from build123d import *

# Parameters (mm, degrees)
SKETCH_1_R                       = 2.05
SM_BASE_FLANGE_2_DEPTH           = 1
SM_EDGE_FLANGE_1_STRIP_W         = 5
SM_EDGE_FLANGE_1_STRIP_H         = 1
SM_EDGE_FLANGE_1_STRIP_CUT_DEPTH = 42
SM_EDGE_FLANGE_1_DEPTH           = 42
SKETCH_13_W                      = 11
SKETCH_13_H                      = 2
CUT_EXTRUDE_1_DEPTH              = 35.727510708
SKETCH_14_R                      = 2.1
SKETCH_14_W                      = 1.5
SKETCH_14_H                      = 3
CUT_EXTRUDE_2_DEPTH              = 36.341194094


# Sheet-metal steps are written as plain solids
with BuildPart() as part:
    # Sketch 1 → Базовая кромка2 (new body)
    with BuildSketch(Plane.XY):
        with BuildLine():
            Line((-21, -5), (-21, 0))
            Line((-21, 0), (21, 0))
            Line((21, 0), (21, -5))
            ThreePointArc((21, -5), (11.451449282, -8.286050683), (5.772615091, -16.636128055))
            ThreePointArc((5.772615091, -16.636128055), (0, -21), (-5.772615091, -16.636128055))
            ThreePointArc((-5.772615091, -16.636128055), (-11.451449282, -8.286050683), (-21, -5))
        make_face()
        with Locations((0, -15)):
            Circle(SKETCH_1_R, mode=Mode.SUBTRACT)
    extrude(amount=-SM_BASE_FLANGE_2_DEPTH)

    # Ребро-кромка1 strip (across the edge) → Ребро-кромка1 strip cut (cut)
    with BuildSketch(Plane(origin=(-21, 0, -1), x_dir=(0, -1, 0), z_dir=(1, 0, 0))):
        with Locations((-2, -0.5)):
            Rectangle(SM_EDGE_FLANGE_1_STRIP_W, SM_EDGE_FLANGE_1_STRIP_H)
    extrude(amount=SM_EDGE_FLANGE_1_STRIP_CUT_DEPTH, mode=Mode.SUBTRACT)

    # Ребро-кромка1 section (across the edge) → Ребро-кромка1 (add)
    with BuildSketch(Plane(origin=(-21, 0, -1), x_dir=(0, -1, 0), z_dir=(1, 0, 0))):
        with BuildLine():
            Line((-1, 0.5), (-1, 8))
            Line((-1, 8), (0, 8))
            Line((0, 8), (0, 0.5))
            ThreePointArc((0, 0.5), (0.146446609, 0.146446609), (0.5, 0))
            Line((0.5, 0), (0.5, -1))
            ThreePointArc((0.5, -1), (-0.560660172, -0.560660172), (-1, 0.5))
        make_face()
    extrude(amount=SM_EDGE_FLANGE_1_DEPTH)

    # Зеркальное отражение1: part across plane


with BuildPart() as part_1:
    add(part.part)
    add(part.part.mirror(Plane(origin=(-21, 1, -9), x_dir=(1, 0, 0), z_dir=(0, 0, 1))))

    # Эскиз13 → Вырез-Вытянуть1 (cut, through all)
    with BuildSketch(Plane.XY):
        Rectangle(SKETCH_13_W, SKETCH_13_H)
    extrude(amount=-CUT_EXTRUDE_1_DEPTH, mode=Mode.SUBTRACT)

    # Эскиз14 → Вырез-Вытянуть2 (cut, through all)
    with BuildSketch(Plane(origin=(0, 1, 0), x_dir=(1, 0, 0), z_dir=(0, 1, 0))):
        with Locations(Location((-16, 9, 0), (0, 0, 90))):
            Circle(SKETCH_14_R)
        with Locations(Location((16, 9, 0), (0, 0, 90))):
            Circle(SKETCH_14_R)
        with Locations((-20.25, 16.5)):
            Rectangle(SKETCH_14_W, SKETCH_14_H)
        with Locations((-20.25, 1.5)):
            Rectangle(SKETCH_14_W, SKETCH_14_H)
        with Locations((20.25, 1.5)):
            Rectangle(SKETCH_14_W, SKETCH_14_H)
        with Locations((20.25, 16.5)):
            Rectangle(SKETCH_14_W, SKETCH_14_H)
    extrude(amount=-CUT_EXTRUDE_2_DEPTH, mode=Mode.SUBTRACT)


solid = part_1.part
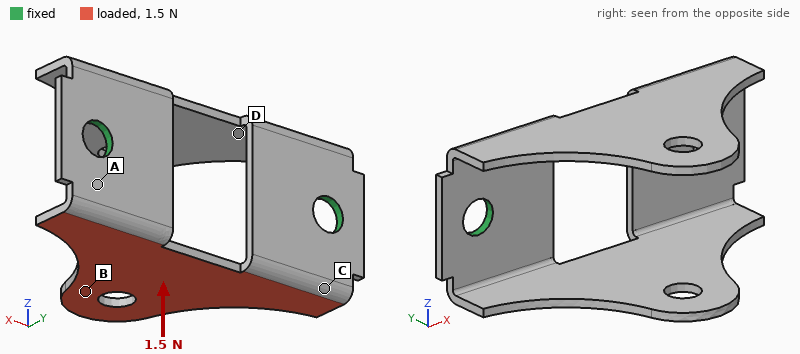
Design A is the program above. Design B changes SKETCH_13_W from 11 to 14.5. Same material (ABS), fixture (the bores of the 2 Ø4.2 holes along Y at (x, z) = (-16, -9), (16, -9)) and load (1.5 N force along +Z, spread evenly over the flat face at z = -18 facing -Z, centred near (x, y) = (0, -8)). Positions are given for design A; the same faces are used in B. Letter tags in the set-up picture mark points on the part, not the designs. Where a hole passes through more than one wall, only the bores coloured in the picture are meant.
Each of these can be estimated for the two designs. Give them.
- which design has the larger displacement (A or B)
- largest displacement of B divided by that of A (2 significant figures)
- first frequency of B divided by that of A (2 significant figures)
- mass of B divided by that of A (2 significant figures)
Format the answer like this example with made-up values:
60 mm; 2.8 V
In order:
B; 1.1; 0.94; 0.95
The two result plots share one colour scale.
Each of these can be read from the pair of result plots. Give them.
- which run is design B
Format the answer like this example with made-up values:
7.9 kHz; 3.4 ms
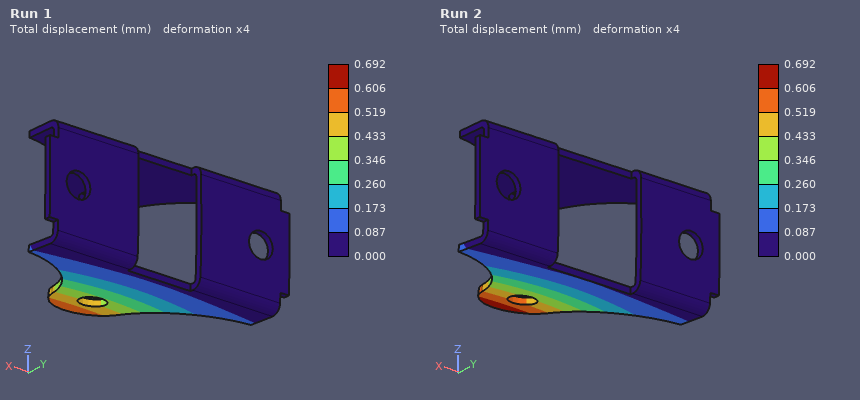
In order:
Run 2
